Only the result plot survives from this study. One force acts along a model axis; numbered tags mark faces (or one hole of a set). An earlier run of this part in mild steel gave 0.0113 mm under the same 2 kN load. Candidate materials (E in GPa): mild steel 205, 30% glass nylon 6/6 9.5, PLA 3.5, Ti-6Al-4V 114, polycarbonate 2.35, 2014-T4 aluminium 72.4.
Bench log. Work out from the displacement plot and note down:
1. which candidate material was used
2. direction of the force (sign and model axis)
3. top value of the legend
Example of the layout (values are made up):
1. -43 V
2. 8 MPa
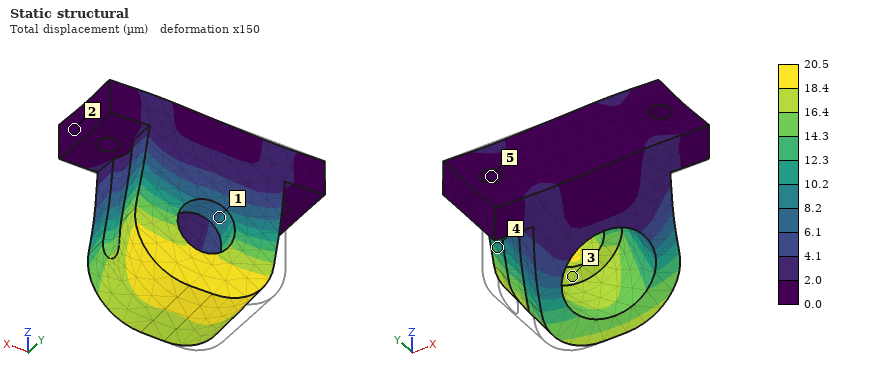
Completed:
1. Ti-6Al-4V
2. +X
3. 20.5 µm
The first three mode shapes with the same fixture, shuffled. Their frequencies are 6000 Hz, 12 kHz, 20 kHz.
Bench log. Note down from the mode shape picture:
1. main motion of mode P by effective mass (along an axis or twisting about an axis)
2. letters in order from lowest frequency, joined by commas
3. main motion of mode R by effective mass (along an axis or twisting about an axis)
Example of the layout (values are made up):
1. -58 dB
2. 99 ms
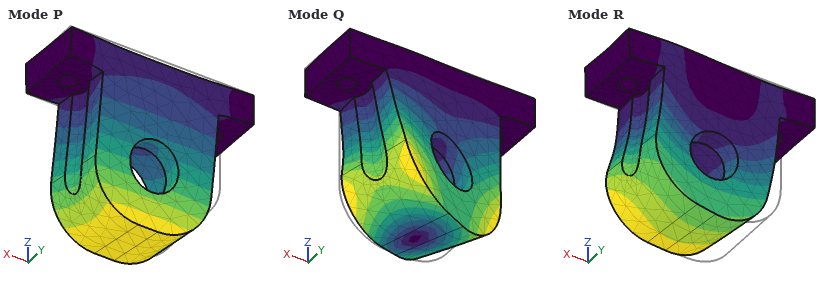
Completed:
1. along Y
2. P, R, Q
3. along X
